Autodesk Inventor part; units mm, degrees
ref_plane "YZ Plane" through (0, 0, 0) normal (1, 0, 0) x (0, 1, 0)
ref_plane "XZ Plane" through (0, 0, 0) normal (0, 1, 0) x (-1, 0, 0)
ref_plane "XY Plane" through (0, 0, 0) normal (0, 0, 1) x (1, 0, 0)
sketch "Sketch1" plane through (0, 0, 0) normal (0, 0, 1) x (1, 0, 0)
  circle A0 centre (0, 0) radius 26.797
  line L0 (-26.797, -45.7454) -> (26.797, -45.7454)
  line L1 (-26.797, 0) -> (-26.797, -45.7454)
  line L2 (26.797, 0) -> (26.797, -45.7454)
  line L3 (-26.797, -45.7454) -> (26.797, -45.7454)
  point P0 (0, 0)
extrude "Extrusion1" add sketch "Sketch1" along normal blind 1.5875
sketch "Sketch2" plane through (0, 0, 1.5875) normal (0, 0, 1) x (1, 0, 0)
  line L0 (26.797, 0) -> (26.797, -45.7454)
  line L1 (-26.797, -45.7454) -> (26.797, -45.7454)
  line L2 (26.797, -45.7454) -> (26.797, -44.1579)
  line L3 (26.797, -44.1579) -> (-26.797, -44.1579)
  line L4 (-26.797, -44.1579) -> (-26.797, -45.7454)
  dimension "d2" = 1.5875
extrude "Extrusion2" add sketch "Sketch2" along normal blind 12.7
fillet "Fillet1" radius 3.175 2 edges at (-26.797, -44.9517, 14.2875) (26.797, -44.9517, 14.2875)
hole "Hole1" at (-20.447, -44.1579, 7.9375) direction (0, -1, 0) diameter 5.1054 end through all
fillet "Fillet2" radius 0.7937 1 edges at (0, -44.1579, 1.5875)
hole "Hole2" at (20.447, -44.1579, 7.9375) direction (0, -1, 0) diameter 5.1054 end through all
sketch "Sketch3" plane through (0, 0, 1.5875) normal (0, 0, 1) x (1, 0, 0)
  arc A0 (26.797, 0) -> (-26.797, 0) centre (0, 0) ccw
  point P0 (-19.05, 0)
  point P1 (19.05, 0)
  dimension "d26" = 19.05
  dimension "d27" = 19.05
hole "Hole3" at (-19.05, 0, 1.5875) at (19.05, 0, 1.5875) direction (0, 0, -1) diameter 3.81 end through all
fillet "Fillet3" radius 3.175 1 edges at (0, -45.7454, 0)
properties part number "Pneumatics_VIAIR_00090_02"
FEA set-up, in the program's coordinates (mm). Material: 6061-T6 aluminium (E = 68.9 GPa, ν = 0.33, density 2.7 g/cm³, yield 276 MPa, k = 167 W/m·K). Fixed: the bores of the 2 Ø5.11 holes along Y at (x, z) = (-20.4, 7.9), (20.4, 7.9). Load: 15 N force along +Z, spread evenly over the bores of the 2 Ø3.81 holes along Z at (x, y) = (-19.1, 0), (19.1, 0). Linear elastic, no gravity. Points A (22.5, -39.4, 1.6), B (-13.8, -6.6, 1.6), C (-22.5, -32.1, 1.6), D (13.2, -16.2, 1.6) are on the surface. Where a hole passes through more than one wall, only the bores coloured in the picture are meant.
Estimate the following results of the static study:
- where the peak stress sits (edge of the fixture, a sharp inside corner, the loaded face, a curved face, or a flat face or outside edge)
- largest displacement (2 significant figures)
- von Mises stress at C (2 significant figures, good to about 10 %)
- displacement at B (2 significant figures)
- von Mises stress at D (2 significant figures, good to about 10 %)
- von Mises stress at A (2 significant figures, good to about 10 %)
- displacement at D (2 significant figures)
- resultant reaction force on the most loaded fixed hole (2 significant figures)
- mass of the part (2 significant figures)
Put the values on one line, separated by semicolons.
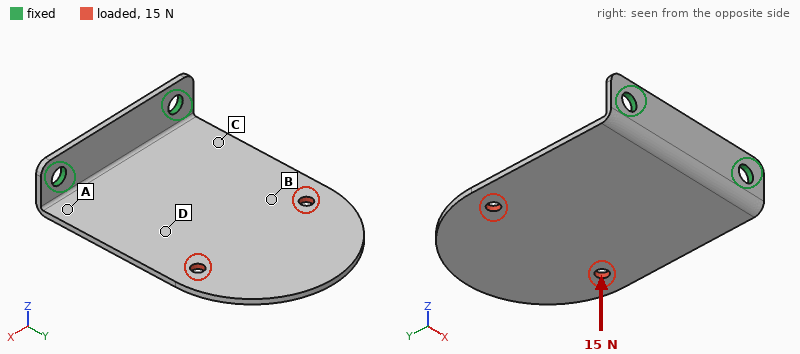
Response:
a curved face; 0.96 mm; 20 MPa; 0.43 mm; 10 MPa; 24 MPa; 0.29 mm; 7.9 N; 18 g
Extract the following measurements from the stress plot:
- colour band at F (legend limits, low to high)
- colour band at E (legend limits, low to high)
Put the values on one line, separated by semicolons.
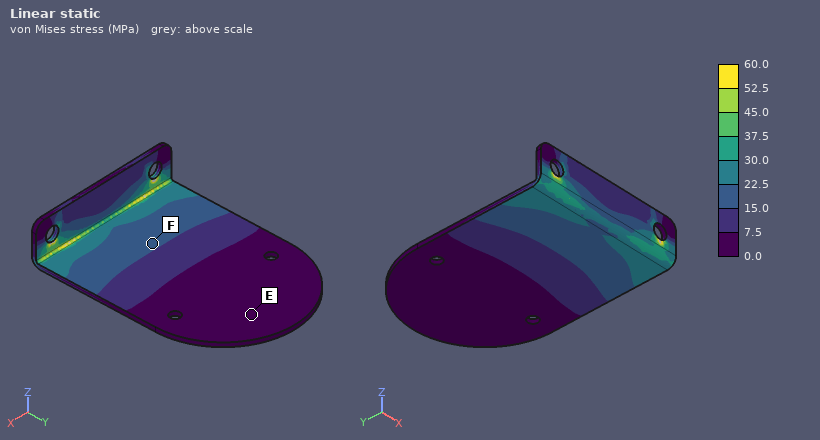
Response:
15.0 to 22.5 MPa; 0.0 to 7.5 MPa
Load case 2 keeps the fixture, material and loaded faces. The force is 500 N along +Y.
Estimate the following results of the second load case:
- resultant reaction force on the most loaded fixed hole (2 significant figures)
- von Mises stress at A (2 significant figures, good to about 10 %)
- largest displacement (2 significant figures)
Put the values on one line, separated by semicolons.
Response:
250 N; 21 MPa; 0.62 mm
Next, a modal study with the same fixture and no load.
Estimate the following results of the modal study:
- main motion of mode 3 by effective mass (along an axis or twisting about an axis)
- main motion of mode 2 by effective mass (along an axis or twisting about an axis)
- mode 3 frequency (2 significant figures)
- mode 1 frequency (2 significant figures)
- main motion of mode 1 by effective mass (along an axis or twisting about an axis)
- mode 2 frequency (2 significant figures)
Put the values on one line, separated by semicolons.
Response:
along Z; twisting about Y; 1500 Hz; 250 Hz; along Z; 890 Hz
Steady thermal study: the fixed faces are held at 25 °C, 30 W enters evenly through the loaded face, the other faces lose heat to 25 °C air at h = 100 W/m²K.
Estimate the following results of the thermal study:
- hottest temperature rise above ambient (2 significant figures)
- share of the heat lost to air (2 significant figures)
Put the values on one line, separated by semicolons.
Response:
59 K; 73 %
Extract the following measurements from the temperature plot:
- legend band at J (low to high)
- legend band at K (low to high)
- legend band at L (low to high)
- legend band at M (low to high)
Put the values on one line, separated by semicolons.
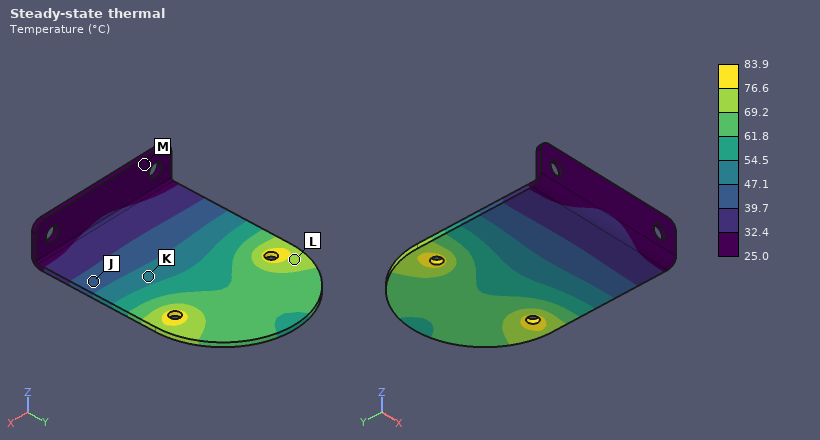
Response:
39.7 to 47.1 °C; 47.1 to 54.5 °C; 69.2 to 76.6 °C; 25.0 to 32.4 °C
